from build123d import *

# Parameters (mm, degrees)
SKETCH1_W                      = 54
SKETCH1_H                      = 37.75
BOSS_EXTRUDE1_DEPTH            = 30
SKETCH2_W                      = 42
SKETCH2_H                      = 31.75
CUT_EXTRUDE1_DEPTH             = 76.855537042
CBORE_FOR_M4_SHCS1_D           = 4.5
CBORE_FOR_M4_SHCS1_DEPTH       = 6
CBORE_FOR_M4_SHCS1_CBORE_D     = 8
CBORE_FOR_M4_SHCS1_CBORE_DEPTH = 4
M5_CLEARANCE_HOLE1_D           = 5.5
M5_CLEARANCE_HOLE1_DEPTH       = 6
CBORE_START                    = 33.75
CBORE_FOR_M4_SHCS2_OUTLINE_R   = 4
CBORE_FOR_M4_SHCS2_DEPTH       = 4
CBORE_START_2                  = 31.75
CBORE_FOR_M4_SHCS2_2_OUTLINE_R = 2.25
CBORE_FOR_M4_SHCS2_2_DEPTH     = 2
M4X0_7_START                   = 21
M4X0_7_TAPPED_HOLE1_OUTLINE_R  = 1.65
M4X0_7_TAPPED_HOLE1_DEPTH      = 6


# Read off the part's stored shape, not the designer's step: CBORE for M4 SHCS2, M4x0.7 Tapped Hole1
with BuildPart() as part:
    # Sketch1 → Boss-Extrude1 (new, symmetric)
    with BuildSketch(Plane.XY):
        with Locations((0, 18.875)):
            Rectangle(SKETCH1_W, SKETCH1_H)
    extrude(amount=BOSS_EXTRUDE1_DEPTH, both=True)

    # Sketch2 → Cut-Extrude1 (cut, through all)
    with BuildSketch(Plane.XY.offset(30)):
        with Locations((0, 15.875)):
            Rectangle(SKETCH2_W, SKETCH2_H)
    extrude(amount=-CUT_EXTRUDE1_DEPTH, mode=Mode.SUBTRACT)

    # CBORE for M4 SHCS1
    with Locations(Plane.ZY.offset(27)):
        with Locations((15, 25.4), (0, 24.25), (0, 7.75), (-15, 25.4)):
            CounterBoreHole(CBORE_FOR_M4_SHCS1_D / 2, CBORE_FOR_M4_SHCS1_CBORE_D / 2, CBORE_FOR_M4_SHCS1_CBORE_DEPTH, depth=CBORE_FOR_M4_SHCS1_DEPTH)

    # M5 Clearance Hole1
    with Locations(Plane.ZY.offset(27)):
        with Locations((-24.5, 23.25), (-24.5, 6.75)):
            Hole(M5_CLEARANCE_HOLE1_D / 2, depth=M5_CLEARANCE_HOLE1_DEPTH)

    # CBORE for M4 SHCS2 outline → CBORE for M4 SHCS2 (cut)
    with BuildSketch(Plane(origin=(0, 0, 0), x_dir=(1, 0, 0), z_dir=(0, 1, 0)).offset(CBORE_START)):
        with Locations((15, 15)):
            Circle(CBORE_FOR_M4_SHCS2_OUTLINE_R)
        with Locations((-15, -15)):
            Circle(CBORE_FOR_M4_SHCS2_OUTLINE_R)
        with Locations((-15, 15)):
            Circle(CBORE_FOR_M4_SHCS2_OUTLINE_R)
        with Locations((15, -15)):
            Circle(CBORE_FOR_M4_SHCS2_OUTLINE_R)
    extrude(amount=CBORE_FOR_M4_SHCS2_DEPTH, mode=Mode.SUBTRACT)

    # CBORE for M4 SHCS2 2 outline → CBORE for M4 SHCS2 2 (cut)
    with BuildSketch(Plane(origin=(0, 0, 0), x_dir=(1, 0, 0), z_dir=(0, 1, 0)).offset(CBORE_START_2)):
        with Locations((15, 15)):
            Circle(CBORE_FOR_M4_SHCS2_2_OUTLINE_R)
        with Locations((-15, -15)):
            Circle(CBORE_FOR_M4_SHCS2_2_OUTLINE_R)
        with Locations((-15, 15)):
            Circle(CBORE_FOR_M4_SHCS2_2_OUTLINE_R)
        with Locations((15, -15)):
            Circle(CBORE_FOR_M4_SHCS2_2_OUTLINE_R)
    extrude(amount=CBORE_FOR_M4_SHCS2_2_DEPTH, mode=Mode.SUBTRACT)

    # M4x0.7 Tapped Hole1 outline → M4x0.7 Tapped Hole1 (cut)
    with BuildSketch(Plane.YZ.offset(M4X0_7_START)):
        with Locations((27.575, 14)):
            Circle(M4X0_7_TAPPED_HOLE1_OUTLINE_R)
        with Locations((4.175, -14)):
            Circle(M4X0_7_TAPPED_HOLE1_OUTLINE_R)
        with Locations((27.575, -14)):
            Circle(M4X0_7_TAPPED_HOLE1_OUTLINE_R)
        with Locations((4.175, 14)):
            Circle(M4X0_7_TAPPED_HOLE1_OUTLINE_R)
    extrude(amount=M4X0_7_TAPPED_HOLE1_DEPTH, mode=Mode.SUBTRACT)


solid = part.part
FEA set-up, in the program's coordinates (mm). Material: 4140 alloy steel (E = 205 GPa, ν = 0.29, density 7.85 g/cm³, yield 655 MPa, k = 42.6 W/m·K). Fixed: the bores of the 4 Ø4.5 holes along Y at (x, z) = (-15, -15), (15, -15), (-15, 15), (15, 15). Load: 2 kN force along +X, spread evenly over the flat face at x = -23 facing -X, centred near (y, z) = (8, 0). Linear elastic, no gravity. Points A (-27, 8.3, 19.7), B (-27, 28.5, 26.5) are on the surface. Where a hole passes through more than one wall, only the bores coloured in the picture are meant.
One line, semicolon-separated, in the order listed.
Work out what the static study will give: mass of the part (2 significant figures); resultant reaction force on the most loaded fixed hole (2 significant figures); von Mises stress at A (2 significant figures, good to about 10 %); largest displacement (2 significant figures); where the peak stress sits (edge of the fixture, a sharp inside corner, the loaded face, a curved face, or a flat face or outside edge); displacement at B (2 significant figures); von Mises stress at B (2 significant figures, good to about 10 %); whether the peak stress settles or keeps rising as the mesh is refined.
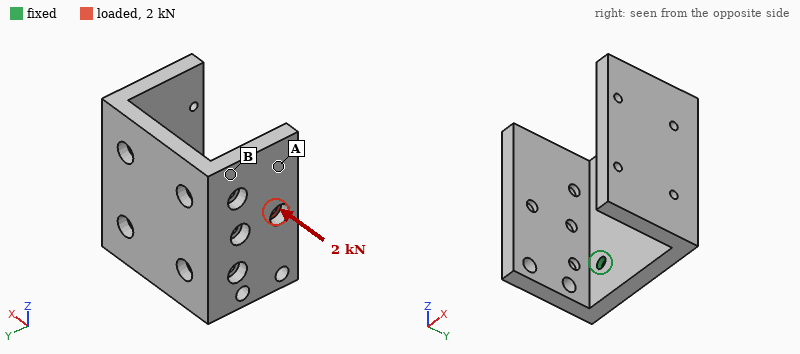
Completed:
310 g; 2.7 kN; 36 MPa; 0.24 mm; edge of the fixture; 0.043 mm; 130 MPa; keeps rising
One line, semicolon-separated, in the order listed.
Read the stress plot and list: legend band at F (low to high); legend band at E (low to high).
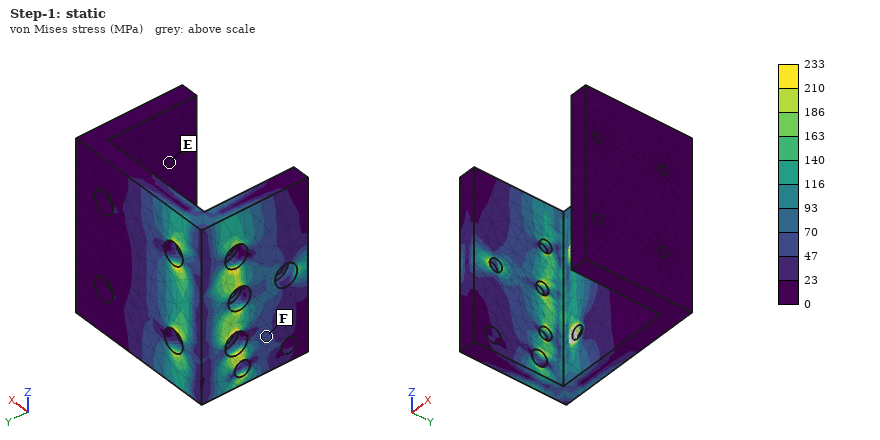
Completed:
47 to 70 MPa; 0 to 23 MPa
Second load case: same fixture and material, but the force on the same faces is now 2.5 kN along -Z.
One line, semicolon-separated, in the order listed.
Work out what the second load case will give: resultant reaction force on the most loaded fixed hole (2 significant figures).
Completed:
2.6 kN
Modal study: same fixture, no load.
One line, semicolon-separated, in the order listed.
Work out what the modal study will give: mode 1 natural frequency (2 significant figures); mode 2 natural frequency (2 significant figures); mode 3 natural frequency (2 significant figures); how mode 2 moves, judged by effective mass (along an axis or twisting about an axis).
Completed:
2500 Hz; 2600 Hz; 4800 Hz; along X
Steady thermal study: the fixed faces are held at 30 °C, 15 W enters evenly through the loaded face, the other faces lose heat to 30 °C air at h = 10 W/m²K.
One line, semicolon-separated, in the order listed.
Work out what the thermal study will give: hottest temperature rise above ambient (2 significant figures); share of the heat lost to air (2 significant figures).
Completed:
75 K; 15 %
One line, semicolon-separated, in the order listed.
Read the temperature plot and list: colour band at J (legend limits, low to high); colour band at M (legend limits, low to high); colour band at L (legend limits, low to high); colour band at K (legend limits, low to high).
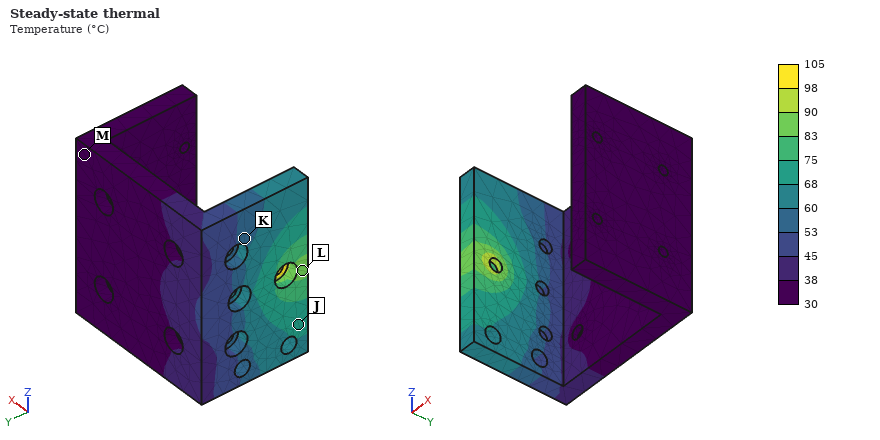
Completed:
68 to 75 °C; 30 to 38 °C; 83 to 90 °C; 53 to 60 °C
